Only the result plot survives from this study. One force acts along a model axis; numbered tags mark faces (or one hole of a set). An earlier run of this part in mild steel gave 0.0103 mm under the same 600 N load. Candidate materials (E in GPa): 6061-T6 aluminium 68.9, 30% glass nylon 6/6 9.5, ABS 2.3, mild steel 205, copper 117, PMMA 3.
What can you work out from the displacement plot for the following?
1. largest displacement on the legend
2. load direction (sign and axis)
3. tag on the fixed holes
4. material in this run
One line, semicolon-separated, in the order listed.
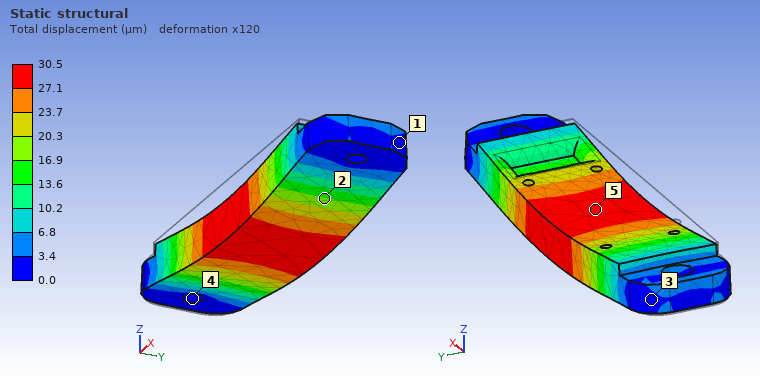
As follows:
30.5 µm; -Z; 4; 6061-T6 aluminium
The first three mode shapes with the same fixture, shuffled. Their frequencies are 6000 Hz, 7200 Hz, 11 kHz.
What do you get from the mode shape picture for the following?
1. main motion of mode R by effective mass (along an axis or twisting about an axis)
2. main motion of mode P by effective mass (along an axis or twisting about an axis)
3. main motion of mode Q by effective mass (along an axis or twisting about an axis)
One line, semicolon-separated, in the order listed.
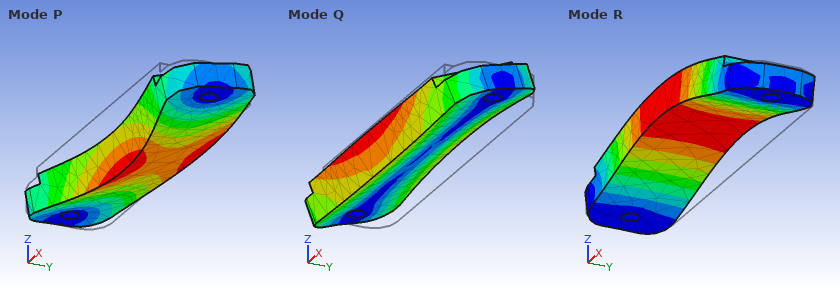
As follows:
along Z; along Y; along Y
